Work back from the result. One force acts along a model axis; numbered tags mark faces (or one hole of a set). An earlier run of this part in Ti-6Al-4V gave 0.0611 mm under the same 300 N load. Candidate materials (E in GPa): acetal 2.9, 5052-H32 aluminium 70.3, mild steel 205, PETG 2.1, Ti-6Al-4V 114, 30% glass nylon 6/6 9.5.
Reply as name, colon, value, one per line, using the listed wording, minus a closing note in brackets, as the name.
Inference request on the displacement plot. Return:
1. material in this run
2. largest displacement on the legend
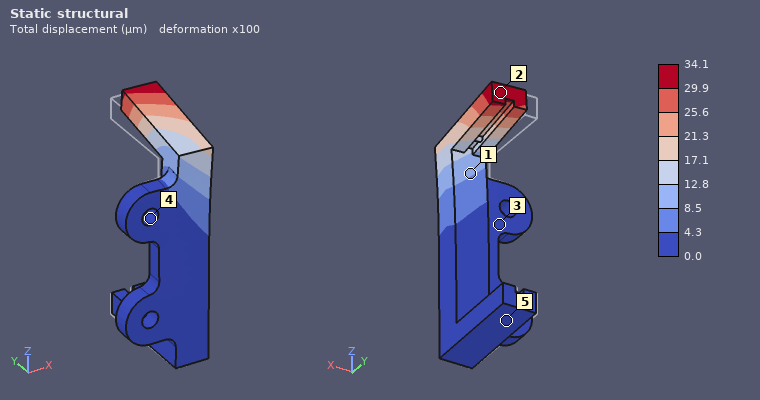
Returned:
material in this run: mild steel
largest displacement on the legend: 34.1 µm
